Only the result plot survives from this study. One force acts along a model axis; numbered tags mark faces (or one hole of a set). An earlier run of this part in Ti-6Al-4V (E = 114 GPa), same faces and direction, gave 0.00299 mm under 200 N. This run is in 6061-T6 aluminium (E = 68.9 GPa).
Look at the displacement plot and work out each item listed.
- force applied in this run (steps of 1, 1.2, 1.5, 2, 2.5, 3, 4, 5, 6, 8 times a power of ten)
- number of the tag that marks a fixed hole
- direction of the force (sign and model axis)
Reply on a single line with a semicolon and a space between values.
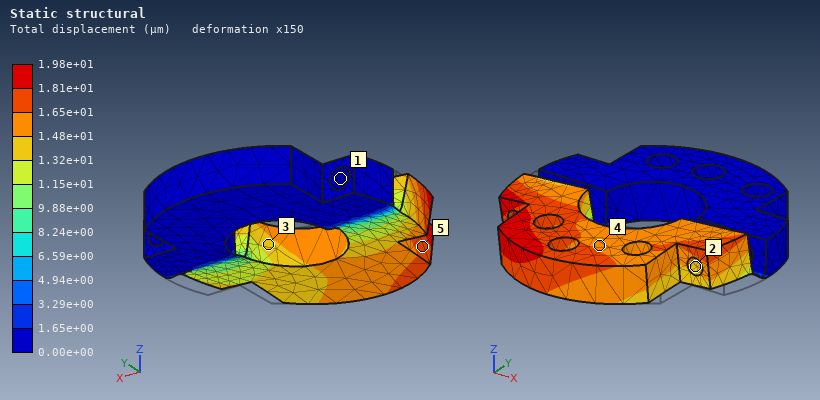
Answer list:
800 N; 1; -X
